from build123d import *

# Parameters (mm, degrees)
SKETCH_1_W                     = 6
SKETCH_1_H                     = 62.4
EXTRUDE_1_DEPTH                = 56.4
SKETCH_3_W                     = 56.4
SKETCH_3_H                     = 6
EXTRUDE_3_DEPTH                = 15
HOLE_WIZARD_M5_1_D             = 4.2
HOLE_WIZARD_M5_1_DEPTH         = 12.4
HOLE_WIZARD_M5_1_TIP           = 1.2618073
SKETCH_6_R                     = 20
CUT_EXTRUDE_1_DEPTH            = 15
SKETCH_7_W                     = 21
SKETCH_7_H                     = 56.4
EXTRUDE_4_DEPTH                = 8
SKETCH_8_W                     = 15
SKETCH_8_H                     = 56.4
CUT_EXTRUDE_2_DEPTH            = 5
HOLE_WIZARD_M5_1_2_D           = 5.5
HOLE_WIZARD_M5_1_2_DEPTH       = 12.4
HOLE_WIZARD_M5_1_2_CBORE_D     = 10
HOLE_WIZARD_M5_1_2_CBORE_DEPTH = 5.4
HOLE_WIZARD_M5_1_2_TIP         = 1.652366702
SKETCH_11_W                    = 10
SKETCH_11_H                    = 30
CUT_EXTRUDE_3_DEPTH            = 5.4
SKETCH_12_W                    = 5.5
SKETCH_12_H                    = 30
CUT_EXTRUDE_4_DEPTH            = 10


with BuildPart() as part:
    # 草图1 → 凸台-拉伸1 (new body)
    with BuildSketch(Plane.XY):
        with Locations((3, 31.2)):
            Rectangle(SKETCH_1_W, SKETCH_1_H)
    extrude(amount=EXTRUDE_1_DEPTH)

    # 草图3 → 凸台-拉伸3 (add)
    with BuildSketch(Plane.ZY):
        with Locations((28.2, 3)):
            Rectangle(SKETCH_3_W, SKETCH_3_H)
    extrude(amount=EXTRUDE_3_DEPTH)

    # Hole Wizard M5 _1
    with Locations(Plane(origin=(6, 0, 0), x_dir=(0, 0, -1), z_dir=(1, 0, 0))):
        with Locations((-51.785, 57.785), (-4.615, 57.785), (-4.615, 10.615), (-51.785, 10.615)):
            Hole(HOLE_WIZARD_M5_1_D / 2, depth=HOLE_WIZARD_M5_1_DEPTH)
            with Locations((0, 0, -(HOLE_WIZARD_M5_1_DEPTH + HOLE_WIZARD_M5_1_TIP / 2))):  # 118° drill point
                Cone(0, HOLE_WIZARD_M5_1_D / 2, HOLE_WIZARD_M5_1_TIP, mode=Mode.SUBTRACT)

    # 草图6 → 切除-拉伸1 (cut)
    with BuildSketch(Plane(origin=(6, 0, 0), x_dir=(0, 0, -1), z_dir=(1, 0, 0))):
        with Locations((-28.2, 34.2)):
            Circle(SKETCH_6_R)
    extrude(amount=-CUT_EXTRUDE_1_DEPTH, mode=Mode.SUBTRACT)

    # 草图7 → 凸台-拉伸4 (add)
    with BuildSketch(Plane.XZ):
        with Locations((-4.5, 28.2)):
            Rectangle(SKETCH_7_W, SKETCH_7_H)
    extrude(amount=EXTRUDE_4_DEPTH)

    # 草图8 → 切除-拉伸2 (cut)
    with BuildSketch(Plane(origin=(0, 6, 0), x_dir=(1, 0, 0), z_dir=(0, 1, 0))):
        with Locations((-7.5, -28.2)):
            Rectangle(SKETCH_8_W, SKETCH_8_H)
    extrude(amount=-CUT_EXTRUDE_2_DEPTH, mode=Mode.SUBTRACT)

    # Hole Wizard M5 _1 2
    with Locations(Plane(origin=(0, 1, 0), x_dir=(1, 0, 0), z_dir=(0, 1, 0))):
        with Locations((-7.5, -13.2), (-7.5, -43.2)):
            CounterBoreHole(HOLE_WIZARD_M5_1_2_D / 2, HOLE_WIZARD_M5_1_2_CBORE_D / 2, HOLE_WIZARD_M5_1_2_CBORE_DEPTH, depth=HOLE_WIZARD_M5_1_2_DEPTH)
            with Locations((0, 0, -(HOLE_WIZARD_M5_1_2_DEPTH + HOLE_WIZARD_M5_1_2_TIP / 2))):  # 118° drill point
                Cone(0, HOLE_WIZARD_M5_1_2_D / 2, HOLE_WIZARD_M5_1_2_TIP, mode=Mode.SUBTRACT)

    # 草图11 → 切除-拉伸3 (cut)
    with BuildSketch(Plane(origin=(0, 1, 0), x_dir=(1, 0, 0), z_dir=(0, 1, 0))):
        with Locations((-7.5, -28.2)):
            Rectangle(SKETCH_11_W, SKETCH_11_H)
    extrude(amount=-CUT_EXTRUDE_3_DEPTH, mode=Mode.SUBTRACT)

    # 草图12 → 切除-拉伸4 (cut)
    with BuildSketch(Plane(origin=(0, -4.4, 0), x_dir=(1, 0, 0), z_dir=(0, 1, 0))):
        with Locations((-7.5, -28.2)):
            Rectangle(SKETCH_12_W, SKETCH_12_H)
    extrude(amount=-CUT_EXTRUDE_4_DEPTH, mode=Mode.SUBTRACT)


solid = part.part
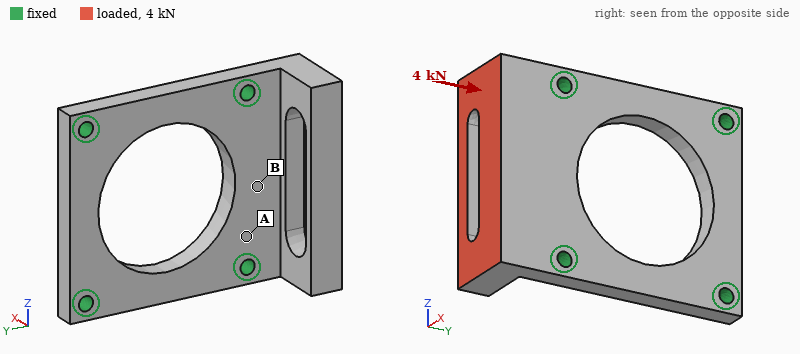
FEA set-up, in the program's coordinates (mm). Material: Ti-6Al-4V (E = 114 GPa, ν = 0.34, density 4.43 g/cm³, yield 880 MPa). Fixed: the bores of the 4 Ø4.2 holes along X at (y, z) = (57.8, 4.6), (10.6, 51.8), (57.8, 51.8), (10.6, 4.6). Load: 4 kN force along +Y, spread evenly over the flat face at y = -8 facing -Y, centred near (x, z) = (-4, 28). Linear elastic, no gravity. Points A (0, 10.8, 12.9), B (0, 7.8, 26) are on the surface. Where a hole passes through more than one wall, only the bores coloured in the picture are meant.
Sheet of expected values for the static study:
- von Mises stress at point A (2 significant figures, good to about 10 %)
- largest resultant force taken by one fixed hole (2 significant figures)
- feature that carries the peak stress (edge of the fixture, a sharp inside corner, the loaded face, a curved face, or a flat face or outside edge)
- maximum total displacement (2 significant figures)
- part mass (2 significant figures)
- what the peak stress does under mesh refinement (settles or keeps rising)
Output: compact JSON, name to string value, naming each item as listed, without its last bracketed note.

{"von Mises stress at point A": "69 MPa", "largest resultant force taken by one fixed hole": "2.0 kN", "feature that carries the peak stress": "edge of the fixture", "maximum total displacement": "0.12 mm", "part mass": "92 g", "what the peak stress does under mesh refinement": "keeps rising"}
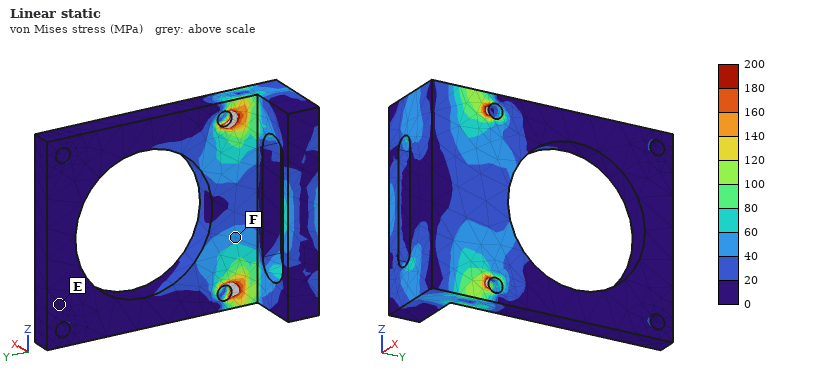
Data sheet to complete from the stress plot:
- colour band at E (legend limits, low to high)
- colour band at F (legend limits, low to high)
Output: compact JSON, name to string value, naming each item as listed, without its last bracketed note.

{"colour band at E": "0 to 20 MPa", "colour band at F": "40 to 60 MPa"}
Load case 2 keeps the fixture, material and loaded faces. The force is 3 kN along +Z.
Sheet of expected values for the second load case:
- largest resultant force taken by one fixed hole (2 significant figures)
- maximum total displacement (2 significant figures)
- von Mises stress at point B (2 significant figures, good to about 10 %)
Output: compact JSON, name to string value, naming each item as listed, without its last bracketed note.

{"largest resultant force taken by one fixed hole": "1.9 kN", "maximum total displacement": "22 µm", "von Mises stress at point B": "14 MPa"}
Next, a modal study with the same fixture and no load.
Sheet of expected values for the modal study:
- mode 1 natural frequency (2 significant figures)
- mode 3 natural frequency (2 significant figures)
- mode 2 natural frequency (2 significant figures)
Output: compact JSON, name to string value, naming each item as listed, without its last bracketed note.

{"mode 1 natural frequency": "4900 Hz", "mode 3 natural frequency": "11 kHz", "mode 2 natural frequency": "8400 Hz"}
